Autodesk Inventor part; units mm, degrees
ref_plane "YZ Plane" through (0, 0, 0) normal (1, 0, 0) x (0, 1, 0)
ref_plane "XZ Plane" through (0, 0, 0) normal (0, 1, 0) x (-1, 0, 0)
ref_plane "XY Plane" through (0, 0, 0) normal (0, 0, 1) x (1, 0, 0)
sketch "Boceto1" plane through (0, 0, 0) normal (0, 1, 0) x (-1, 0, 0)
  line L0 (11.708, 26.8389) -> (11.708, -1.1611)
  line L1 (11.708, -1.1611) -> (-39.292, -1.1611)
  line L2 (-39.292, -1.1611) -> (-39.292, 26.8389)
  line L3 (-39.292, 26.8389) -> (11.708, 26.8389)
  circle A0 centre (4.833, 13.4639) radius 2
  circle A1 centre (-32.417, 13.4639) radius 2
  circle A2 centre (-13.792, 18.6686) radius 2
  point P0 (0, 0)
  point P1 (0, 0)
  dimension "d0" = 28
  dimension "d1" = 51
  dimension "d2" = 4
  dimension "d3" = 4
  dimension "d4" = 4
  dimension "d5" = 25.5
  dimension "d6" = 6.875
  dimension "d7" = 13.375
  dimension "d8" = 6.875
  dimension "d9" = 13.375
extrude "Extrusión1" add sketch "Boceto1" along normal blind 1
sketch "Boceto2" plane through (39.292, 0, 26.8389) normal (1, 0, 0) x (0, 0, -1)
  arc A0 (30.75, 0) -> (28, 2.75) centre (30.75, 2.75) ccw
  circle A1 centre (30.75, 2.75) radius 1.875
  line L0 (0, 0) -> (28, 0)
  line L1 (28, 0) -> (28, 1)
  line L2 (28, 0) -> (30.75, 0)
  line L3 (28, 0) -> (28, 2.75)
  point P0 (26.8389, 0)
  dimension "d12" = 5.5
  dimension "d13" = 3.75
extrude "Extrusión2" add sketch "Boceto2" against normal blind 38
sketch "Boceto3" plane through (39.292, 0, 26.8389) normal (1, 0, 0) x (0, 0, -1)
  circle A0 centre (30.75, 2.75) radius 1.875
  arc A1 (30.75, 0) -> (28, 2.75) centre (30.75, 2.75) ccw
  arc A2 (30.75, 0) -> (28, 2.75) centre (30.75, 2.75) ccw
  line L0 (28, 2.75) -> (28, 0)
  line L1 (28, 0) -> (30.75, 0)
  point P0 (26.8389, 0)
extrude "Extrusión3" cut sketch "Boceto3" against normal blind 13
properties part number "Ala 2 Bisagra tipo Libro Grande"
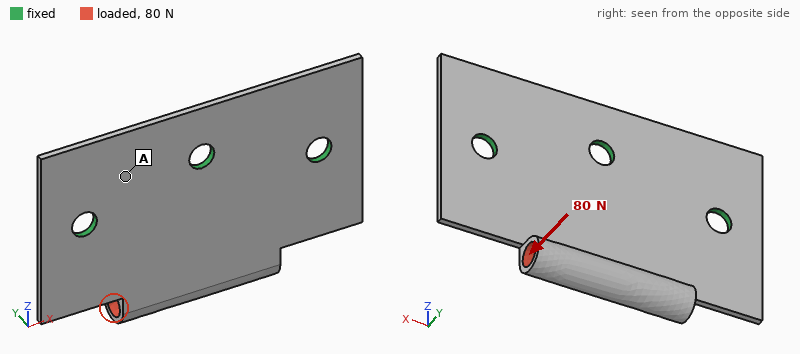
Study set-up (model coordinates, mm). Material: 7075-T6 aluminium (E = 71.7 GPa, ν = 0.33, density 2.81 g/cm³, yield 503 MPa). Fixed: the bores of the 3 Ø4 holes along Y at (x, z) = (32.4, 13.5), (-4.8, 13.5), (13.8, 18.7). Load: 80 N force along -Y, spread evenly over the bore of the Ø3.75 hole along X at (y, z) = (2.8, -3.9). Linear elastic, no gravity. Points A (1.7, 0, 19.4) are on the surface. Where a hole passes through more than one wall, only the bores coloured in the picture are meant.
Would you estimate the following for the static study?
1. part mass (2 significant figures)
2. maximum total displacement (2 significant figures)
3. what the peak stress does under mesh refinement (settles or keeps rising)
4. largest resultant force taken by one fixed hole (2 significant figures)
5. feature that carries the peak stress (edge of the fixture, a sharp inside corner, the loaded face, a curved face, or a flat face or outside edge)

4.9 g
0.67 mm
keeps rising
43 N
edge of the fixture
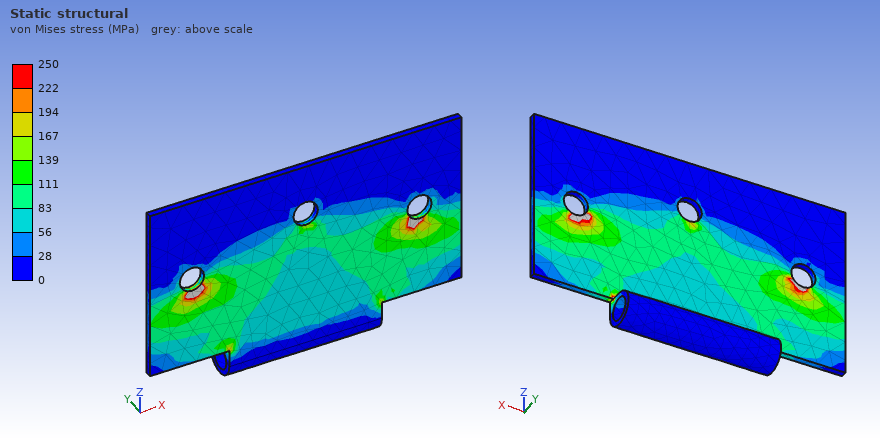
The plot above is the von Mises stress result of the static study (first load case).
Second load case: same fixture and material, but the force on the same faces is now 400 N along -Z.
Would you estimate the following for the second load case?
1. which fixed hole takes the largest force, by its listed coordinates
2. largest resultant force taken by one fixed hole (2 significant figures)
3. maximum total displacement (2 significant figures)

(13.8, 18.7)
210 N
0.66 mm
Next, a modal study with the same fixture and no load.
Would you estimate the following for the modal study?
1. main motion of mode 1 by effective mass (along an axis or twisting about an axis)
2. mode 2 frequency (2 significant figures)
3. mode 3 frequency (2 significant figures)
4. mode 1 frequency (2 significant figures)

along Y
4400 Hz
6400 Hz
1700 Hz
